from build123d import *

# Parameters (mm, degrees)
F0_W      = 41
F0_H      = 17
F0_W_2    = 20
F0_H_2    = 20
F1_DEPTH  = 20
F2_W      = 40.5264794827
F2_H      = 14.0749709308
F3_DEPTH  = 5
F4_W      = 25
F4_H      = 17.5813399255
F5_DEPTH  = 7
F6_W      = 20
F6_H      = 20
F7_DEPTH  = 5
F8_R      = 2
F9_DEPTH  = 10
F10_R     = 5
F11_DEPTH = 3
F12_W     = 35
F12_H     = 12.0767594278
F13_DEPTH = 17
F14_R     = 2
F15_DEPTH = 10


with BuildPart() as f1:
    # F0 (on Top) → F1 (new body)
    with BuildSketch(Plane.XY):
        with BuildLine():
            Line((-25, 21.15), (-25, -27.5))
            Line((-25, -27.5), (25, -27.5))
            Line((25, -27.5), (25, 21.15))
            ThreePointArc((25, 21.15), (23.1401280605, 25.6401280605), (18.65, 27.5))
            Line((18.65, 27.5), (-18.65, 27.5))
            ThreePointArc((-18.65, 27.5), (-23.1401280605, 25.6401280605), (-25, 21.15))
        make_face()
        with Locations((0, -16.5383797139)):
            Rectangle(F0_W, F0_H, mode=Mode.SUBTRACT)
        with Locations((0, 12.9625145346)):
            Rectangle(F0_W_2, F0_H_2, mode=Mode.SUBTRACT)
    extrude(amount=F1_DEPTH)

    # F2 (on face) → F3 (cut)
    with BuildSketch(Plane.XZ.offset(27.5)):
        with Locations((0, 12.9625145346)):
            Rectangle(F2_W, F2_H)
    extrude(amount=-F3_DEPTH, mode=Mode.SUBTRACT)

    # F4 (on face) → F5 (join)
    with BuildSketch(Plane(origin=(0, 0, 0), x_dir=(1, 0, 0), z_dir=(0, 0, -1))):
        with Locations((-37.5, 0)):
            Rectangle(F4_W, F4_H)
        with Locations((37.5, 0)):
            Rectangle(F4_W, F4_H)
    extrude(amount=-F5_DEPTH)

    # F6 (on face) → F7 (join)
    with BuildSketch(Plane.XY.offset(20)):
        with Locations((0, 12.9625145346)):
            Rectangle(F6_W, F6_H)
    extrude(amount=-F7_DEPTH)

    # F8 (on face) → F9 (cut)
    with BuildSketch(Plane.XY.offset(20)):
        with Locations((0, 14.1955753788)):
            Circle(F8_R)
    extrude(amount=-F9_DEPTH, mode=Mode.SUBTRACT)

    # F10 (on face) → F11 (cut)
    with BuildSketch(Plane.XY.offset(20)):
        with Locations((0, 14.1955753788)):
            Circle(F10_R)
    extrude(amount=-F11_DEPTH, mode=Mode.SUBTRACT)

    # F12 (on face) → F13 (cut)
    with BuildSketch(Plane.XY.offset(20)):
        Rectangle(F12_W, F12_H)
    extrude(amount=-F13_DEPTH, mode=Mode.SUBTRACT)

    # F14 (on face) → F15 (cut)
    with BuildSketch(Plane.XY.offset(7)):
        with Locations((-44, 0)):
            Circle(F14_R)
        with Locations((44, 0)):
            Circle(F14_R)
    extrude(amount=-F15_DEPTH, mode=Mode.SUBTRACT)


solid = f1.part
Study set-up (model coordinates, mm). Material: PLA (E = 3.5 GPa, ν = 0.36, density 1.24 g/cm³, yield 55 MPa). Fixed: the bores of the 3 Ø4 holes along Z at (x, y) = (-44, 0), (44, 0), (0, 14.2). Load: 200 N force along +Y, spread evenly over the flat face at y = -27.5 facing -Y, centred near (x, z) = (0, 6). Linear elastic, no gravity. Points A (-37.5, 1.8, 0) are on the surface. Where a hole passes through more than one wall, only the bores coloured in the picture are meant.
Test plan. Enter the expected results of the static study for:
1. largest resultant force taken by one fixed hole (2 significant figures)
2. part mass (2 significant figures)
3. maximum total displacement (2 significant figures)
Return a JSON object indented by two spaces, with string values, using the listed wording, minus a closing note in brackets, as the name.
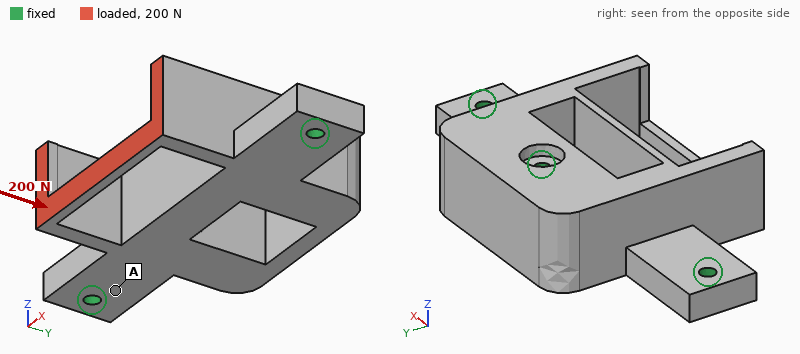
{
  "largest resultant force taken by one fixed hole": "79 N",
  "part mass": "40 g",
  "maximum total displacement": "1.1 mm"
}
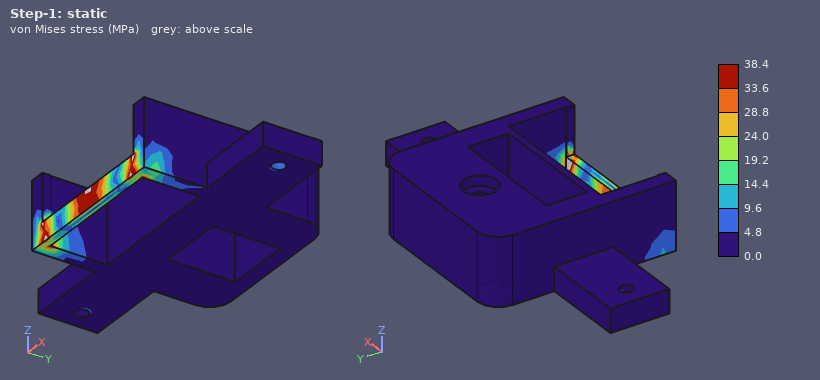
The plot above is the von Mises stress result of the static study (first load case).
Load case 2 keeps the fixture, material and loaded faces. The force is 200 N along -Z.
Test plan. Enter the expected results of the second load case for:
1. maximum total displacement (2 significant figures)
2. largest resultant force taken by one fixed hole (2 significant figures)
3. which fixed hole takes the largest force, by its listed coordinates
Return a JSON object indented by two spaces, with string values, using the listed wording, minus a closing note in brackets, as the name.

{
  "maximum total displacement": "0.80 mm",
  "largest resultant force taken by one fixed hole": "260 N",
  "which fixed hole takes the largest force, by its listed coordinates": "(0, 14.2)"
}
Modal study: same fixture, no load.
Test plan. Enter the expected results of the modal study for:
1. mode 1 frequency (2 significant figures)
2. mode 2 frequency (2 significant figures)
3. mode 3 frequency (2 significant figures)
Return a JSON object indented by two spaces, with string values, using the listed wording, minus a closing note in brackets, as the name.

{
  "mode 1 frequency": "1600 Hz",
  "mode 2 frequency": "2100 Hz",
  "mode 3 frequency": "2100 Hz"
}
